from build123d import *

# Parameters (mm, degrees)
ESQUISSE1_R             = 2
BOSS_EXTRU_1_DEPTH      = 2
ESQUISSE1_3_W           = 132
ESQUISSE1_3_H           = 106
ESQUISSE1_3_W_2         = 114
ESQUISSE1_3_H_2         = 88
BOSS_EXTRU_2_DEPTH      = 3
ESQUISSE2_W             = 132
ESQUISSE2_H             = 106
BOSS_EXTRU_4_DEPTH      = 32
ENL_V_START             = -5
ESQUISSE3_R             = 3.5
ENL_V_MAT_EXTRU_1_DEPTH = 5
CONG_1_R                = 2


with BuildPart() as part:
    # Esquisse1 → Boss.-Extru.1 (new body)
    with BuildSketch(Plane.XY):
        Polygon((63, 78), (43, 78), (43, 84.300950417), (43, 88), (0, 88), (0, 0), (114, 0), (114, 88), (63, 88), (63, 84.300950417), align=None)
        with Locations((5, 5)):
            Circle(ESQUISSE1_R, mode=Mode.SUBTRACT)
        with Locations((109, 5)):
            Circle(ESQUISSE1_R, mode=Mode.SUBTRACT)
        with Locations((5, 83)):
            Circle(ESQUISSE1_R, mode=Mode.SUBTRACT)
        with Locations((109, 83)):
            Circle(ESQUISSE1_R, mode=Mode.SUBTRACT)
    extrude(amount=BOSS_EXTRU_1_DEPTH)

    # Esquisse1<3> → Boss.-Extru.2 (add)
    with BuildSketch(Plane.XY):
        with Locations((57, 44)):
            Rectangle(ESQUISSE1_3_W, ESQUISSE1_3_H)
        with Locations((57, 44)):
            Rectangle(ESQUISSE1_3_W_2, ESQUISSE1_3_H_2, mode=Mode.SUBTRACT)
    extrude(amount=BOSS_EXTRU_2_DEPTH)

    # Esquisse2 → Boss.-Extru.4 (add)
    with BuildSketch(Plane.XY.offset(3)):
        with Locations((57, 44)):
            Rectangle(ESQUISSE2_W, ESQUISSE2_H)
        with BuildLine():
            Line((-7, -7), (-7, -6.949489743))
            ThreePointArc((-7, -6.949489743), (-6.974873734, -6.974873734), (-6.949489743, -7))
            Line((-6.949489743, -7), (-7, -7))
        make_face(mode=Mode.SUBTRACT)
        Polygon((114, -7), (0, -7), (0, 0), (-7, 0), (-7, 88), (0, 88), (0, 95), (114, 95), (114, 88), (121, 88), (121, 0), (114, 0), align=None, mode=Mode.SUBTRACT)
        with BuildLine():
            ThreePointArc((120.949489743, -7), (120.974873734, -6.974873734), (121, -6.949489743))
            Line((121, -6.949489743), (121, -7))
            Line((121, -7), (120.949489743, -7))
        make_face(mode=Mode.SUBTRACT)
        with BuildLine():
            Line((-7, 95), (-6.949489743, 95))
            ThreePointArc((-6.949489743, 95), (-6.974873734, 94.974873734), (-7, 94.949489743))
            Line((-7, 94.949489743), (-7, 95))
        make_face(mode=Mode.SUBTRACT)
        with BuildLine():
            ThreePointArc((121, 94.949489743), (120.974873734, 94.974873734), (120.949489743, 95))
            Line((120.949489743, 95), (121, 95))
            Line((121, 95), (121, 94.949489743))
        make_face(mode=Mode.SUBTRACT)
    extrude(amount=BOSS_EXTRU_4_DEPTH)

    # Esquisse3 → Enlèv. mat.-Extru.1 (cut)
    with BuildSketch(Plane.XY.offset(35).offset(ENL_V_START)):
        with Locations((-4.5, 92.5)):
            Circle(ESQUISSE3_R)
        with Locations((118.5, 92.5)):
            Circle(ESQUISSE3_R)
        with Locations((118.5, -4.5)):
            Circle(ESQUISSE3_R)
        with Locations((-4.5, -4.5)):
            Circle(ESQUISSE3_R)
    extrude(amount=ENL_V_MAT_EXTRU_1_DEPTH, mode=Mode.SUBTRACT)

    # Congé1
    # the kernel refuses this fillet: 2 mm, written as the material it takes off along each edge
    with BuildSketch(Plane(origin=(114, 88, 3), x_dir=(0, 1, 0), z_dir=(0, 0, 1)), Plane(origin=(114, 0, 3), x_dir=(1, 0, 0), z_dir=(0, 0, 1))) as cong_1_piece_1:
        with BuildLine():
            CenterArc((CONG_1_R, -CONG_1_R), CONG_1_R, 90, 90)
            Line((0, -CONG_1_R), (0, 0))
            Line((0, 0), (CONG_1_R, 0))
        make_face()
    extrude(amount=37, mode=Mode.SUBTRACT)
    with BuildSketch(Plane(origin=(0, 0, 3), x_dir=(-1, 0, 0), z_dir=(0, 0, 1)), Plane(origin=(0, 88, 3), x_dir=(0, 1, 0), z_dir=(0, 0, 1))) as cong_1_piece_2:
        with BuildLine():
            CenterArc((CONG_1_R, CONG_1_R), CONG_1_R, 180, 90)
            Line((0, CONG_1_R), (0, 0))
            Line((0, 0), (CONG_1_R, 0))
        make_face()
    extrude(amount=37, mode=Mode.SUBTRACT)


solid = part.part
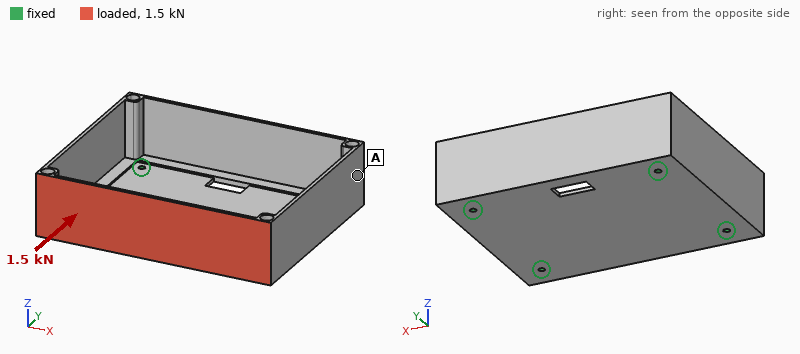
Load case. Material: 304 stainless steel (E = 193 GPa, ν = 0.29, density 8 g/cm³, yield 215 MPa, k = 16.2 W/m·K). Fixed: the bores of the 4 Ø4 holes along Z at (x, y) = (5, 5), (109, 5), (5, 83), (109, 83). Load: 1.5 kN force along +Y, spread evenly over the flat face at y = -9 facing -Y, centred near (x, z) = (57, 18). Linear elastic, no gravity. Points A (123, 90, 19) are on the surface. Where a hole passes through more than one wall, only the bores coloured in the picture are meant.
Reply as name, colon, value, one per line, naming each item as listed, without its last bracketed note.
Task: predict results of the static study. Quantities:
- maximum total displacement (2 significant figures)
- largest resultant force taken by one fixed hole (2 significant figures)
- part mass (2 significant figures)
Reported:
maximum total displacement: 0.40 mm
largest resultant force taken by one fixed hole: 430 N
part mass: 530 g
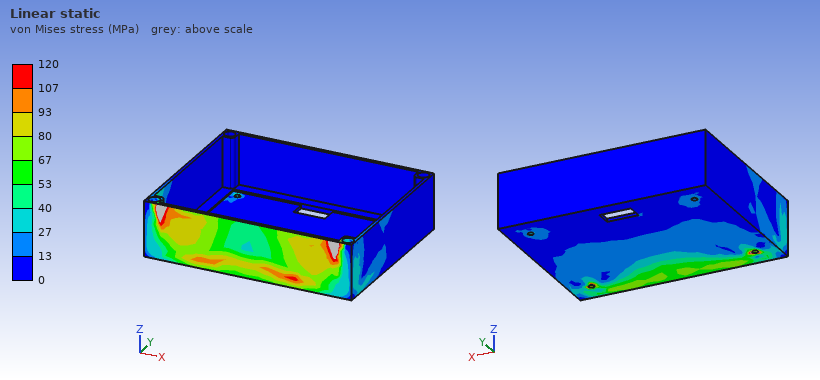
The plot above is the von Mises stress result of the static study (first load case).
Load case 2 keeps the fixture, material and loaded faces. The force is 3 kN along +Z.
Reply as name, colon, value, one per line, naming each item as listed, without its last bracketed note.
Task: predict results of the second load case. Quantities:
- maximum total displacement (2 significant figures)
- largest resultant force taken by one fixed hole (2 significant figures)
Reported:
maximum total displacement: 0.15 mm
largest resultant force taken by one fixed hole: 1.8 kN
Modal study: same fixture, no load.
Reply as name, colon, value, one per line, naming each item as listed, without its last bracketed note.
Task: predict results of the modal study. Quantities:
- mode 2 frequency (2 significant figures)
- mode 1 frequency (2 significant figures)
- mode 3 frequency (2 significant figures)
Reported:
mode 2 frequency: 1500 Hz
mode 1 frequency: 1100 Hz
mode 3 frequency: 1700 Hz
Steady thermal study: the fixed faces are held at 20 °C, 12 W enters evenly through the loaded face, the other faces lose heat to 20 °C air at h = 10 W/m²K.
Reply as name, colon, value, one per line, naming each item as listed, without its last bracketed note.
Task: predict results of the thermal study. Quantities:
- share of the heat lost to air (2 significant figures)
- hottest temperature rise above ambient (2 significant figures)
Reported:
share of the heat lost to air: 57 %
hottest temperature rise above ambient: 68 K
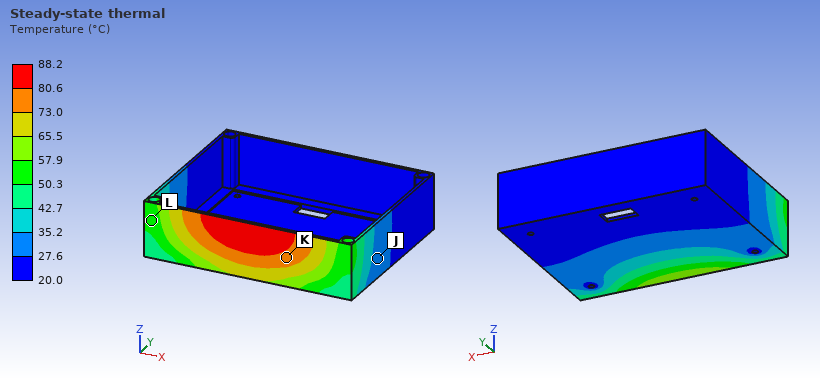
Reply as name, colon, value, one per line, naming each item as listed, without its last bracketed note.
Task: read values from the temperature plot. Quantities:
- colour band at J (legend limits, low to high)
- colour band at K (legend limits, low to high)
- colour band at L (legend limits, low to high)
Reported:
colour band at J: 27.6 to 35.2 °C
colour band at K: 73.0 to 80.6 °C
colour band at L: 50.3 to 57.9 °C
